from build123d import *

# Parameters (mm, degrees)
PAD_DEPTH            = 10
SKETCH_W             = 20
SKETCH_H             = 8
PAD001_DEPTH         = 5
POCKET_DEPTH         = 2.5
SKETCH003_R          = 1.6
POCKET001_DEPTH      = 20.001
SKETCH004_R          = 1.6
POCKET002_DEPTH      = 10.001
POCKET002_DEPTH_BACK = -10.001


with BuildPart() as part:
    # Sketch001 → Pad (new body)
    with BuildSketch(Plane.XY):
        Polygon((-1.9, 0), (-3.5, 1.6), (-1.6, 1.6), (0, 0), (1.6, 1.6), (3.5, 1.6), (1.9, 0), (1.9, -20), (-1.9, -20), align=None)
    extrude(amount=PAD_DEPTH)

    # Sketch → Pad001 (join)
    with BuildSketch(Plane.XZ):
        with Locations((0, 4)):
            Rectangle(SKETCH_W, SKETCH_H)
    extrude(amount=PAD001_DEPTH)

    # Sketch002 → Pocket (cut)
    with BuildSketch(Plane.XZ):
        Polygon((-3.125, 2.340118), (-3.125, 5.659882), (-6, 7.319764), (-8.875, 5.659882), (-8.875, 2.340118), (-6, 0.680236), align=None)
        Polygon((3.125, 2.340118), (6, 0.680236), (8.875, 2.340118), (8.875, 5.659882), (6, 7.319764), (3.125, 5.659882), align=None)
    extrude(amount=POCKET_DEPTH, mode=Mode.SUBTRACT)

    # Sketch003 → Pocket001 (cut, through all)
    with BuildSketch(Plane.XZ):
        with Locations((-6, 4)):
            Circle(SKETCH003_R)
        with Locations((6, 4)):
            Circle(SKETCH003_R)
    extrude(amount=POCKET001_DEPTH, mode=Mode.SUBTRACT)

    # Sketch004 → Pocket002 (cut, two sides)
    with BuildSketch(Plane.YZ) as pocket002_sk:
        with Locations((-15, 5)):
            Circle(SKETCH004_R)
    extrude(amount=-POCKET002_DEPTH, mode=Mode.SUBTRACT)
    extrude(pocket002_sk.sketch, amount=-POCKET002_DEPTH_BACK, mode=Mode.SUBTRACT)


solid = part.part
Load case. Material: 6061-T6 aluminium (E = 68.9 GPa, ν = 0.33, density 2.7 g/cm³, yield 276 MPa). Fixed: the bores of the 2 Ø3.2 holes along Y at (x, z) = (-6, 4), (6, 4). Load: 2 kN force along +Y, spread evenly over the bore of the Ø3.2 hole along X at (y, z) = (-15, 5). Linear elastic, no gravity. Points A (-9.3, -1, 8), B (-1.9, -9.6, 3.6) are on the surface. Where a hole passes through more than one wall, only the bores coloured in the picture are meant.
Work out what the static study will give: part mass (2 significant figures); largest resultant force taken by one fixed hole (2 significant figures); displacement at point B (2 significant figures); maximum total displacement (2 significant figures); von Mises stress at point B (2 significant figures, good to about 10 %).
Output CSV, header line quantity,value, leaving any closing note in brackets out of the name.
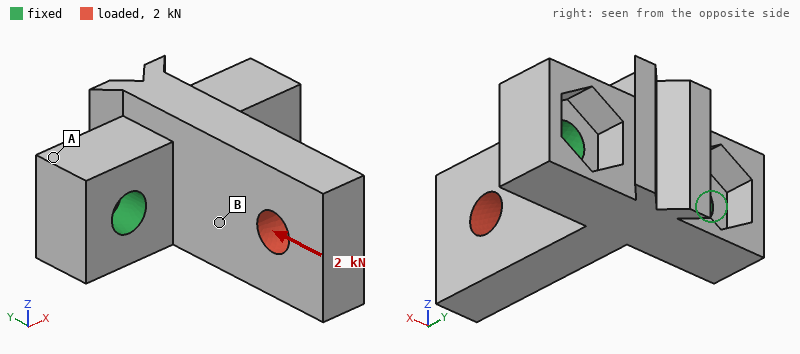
quantity,value
part mass,3.4 g
largest resultant force taken by one fixed hole,1.0 kN
displacement at point B,16 µm
maximum total displacement,37 µm
von Mises stress at point B,59 MPa
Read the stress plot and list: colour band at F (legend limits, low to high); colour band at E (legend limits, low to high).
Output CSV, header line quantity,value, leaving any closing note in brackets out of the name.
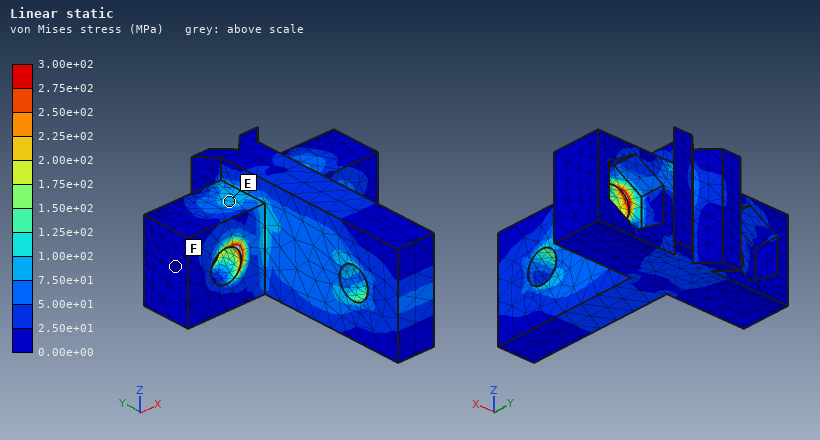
quantity,value
colour band at F,0.00e+00 to 2.50e+01 MPa
colour band at E,7.50e+01 to 1.00e+02 MPa
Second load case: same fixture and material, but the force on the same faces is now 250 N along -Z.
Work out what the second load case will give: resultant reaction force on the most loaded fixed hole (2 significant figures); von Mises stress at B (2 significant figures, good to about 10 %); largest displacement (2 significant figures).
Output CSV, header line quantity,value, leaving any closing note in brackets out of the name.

quantity,value
resultant reaction force on the most loaded fixed hole,130 N
von Mises stress at B,18 MPa
largest displacement,52 µm
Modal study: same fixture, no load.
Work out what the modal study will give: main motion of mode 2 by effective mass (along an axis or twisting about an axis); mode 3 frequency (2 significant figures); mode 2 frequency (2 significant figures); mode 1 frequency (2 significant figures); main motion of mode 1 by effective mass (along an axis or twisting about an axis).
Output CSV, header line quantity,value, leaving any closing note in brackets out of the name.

quantity,value
main motion of mode 2 by effective mass,along Z
mode 3 frequency,31 kHz
mode 2 frequency,12 kHz
mode 1 frequency,11 kHz
main motion of mode 1 by effective mass,along X
